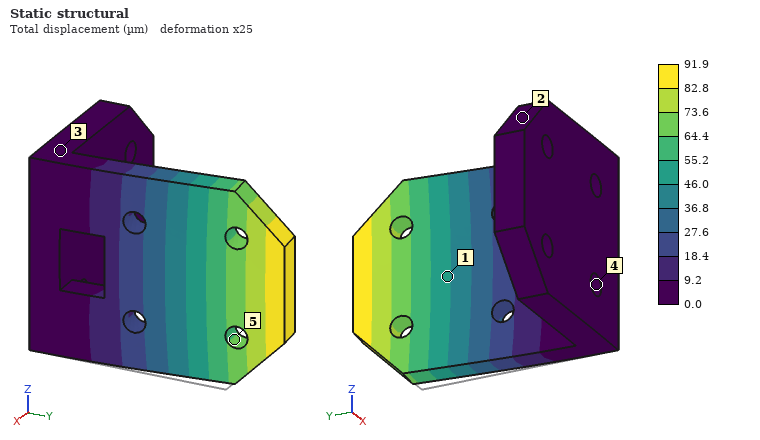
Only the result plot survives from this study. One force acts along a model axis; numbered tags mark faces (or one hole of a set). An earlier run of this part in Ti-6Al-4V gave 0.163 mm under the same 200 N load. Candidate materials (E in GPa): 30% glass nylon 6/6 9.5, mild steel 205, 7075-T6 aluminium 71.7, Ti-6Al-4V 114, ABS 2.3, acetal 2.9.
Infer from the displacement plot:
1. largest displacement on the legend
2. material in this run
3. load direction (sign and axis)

91.9 µm
mild steel
-X
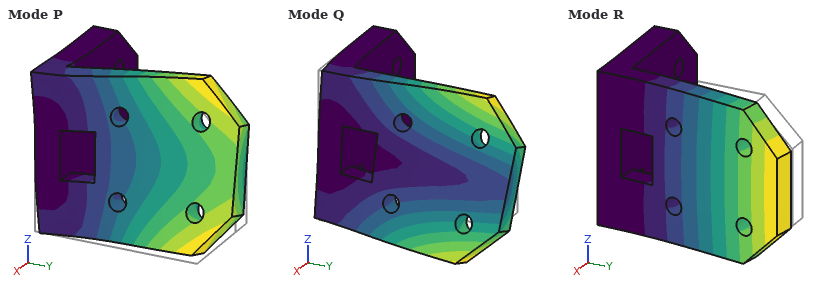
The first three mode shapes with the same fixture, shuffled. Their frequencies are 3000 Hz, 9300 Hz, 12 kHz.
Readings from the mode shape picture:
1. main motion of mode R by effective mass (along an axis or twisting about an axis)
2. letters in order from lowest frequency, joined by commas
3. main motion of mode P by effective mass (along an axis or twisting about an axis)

along X
R, Q, P
along Z
